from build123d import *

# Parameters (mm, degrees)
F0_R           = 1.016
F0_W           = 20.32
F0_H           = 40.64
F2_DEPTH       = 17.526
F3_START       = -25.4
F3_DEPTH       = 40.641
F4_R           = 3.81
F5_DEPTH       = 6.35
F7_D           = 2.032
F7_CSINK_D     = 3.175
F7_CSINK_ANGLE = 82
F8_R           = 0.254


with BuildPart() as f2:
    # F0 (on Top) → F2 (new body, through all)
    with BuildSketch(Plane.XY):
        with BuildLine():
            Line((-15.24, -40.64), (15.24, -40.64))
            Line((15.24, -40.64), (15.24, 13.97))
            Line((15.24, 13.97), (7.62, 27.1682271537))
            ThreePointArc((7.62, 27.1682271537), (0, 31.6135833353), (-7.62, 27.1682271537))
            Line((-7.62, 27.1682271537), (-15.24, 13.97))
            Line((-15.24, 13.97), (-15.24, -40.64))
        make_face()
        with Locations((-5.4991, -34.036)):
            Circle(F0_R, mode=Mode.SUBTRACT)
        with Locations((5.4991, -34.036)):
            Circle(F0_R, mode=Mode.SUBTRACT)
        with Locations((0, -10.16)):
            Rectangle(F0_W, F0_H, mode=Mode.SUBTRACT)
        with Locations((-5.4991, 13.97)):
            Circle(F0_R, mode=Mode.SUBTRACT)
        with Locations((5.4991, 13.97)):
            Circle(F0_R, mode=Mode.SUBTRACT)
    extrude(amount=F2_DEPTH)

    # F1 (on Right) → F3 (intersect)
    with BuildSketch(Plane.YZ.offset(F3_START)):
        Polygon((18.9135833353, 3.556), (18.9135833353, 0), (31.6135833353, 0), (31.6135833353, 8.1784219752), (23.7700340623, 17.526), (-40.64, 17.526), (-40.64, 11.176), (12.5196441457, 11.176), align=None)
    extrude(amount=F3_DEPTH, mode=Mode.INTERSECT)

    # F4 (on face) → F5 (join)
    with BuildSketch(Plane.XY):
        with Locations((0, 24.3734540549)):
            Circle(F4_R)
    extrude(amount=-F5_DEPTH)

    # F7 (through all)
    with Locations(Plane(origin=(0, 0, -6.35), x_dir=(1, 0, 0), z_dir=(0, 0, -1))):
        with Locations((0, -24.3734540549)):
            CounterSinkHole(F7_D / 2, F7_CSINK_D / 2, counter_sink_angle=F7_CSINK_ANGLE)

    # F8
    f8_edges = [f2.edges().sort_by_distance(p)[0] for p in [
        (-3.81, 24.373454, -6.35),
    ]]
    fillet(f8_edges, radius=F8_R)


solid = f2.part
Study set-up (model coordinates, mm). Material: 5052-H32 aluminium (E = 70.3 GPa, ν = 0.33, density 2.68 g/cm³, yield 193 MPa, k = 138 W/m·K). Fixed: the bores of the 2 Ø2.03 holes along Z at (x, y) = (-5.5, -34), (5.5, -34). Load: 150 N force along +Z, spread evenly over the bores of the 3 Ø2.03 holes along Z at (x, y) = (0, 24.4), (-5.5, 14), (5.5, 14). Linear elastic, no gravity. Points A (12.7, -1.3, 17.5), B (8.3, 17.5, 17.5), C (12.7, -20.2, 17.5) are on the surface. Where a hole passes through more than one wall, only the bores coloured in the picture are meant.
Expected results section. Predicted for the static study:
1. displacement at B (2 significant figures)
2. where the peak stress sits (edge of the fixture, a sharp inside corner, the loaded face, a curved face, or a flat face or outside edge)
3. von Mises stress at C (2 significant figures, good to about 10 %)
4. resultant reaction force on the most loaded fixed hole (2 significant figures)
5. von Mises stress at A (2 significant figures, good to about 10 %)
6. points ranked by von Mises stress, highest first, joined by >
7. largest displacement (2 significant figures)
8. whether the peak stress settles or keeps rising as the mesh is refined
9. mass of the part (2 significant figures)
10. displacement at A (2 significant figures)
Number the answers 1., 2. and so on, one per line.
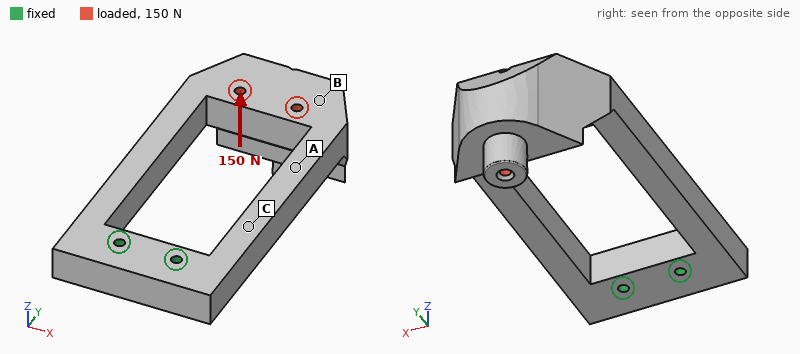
1. 0.58 mm
2. edge of the fixture
3. 88 MPa
4. 75 N
5. 47 MPa
6. C > A > B
7. 0.83 mm
8. keeps rising
9. 28 g
10. 0.29 mm
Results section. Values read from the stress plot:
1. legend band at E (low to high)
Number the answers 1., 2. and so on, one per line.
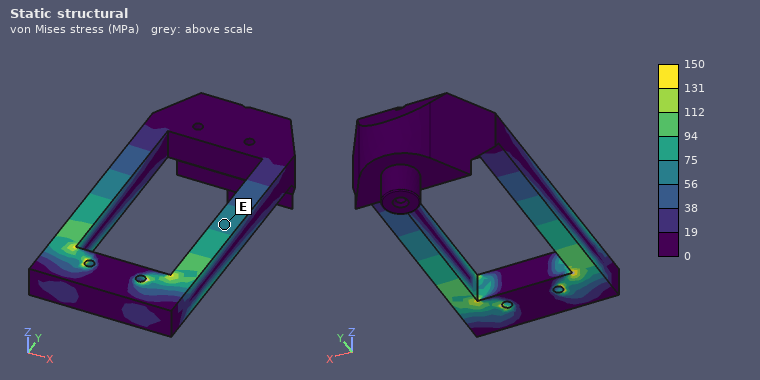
1. 56 to 75 MPa
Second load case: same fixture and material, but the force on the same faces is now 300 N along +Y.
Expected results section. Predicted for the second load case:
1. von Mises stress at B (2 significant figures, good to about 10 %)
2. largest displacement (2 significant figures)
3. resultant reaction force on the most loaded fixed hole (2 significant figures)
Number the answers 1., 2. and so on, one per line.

1. 4.6 MPa
2. 0.26 mm
3. 170 N
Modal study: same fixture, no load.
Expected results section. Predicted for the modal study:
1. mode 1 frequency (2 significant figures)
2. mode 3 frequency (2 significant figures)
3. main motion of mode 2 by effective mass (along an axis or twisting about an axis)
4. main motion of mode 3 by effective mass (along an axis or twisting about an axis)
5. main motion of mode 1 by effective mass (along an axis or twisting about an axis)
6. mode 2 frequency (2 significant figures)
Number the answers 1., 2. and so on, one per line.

1. 590 Hz
2. 2500 Hz
3. along X
4. twisting about Y
5. along Z
6. 1100 Hz
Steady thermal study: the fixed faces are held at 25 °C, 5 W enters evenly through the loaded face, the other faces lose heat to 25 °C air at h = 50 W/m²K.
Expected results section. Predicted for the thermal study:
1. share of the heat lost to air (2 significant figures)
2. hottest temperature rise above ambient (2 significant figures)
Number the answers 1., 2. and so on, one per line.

1. 50 %
2. 17 K
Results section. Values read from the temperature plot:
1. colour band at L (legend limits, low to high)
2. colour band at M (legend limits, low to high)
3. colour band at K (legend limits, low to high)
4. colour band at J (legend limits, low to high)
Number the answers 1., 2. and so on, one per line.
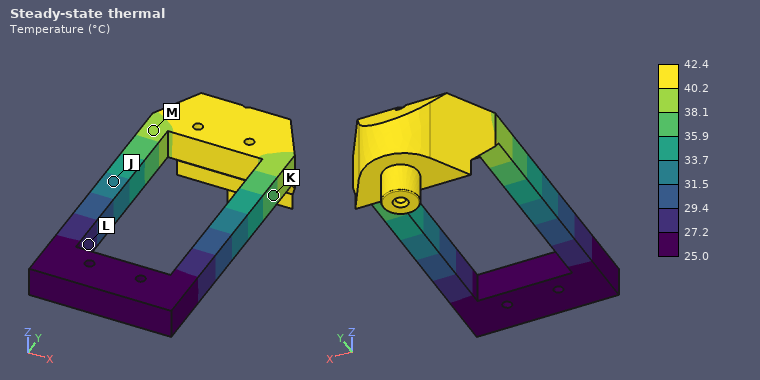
1. 27.2 to 29.4 °C
2. 38.1 to 40.2 °C
3. 35.9 to 38.1 °C
4. 31.5 to 33.7 °C
